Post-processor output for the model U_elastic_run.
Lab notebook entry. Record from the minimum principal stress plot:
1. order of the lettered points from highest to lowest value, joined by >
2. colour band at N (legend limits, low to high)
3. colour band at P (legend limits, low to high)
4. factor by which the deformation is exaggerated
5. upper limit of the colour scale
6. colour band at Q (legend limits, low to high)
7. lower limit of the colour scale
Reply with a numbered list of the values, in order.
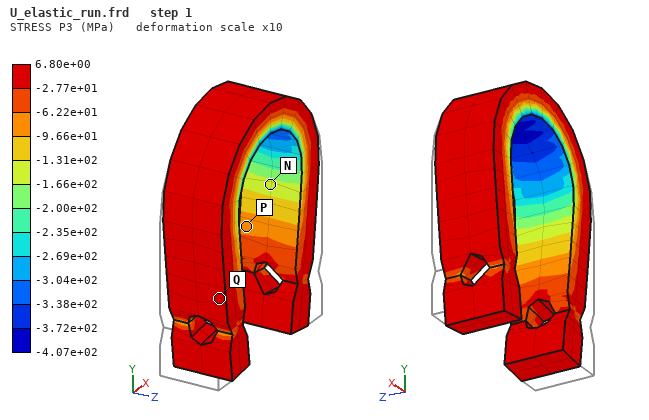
1. Q > P > N
2. -1.66e+02 to -1.31e+02 MPa
3. -9.66e+01 to -6.22e+01 MPa
4. 10
5. 6.80e+00 MPa
6. -2.77e+01 to 6.80e+00 MPa
7. -4.07e+02 MPa
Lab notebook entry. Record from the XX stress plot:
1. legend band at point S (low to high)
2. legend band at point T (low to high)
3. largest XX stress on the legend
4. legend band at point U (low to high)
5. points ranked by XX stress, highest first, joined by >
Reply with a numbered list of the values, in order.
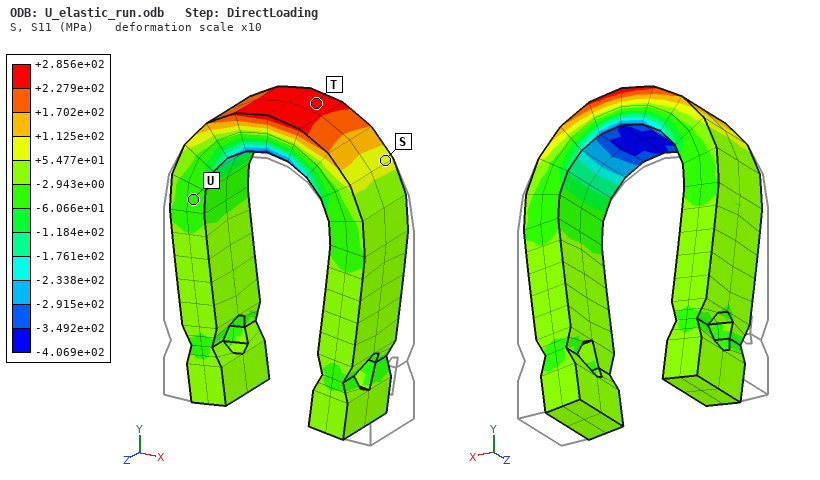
1. +5.477e+01 to +1.125e+02 MPa
2. +2.279e+02 to +2.856e+02 MPa
3. +2.856e+02 MPa
4. -6.066e+01 to -2.943e+00 MPa
5. T > S > U
